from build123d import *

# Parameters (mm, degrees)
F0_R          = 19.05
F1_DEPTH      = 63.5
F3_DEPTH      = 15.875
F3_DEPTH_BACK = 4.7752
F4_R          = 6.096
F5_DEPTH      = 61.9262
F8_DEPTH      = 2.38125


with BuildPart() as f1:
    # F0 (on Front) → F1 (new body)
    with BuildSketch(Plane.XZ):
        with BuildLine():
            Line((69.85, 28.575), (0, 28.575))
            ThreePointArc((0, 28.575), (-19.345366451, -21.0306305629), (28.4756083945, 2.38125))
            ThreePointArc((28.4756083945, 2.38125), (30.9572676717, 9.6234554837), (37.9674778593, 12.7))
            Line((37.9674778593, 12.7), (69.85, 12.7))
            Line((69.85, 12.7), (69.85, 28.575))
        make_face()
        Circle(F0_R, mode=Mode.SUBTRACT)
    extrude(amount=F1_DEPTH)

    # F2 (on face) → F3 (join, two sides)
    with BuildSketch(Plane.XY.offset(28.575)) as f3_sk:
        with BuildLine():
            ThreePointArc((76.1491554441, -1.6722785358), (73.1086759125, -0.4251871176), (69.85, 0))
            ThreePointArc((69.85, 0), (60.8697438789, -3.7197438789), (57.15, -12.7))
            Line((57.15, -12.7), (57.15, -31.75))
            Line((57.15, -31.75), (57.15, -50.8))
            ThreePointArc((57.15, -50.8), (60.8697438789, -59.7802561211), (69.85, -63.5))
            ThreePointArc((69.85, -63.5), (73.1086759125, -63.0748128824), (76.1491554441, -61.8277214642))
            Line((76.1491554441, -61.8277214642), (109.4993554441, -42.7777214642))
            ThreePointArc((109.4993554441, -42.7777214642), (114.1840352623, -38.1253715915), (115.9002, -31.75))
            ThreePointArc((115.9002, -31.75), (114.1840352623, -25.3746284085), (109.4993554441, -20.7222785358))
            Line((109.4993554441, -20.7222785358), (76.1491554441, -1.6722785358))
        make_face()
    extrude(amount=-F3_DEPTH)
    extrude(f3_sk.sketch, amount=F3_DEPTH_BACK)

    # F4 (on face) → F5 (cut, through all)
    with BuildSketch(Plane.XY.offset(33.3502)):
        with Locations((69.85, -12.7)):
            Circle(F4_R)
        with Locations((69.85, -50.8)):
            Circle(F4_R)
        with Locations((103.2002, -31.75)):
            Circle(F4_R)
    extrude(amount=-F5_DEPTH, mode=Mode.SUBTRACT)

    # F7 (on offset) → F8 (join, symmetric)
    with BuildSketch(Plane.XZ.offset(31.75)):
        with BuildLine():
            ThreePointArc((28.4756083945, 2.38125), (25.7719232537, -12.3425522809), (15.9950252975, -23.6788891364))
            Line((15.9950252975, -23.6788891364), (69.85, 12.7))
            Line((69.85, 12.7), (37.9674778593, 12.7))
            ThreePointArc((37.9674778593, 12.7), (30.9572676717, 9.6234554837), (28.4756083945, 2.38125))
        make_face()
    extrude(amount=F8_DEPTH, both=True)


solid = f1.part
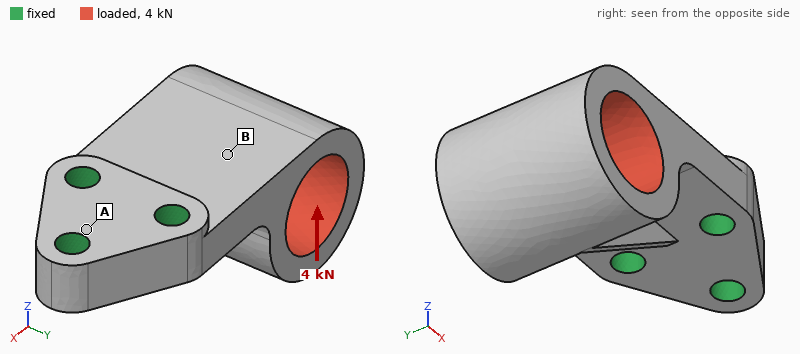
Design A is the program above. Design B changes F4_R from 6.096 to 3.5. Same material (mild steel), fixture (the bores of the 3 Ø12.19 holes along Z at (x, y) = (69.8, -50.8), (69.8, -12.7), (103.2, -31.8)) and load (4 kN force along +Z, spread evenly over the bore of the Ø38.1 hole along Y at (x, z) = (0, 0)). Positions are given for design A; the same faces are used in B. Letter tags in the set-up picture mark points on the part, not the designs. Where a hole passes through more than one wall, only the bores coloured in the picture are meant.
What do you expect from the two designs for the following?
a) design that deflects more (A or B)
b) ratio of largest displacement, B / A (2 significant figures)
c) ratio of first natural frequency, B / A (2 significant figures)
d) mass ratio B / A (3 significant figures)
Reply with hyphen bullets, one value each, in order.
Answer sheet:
- B
- 1.1
- 0.95
- 1.03
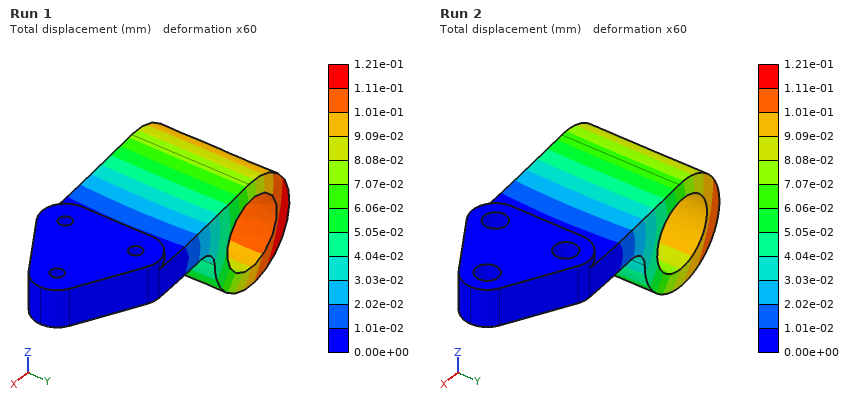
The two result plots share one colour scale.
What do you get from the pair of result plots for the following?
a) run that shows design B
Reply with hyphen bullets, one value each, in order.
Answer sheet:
- Run 1
